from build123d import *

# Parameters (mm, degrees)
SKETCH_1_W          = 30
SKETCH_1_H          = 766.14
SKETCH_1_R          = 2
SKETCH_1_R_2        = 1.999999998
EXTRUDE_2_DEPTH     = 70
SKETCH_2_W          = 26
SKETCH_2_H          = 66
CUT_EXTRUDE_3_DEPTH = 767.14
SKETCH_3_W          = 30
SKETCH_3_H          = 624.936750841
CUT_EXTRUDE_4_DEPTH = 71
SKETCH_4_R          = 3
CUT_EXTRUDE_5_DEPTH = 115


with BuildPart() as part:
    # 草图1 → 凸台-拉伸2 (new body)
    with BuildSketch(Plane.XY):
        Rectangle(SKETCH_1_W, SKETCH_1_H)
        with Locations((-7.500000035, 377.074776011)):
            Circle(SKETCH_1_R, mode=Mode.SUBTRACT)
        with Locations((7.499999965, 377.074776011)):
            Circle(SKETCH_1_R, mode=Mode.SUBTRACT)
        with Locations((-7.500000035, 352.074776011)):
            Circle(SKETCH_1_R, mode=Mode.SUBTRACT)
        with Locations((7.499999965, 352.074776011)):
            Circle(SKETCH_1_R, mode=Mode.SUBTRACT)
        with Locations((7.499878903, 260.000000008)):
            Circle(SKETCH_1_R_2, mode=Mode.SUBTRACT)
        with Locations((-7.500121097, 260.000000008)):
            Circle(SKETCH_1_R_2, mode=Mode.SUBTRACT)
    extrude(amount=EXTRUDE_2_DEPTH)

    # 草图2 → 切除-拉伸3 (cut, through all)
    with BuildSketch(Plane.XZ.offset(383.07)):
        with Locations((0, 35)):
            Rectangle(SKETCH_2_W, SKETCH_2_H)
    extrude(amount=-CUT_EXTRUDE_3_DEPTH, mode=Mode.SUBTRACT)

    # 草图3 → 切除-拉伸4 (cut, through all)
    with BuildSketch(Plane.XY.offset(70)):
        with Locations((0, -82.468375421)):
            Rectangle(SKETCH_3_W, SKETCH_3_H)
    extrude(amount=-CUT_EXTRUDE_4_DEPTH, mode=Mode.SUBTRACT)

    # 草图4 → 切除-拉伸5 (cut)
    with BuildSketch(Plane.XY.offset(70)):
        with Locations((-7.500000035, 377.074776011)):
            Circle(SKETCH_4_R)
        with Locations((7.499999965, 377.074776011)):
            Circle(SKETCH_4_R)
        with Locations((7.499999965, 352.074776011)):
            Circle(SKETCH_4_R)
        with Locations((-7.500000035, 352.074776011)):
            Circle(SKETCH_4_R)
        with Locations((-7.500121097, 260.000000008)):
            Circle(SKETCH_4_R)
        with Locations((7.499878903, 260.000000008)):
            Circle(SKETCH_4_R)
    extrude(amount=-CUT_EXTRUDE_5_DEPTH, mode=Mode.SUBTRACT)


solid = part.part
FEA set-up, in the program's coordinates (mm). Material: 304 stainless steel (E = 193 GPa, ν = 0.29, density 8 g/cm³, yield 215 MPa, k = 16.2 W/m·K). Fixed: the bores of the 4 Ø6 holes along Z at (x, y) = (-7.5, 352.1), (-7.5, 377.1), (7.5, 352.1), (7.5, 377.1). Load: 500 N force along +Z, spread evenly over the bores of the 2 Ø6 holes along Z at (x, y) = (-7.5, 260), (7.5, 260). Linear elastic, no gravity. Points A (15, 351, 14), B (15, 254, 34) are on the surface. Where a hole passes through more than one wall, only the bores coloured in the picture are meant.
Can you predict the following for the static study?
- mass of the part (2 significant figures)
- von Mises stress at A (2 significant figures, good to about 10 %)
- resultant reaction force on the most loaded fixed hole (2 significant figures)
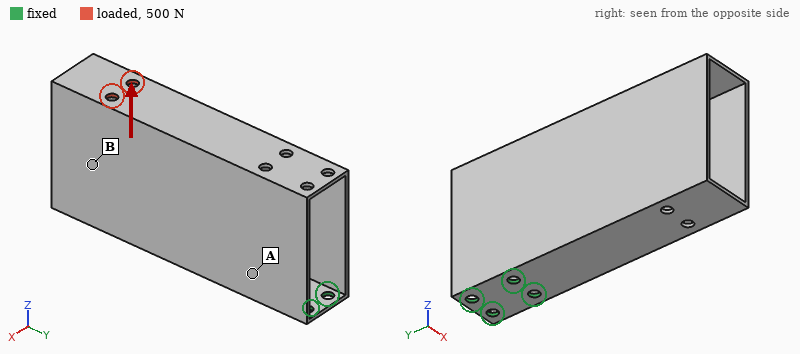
460 g
27 MPa
1.1 kN
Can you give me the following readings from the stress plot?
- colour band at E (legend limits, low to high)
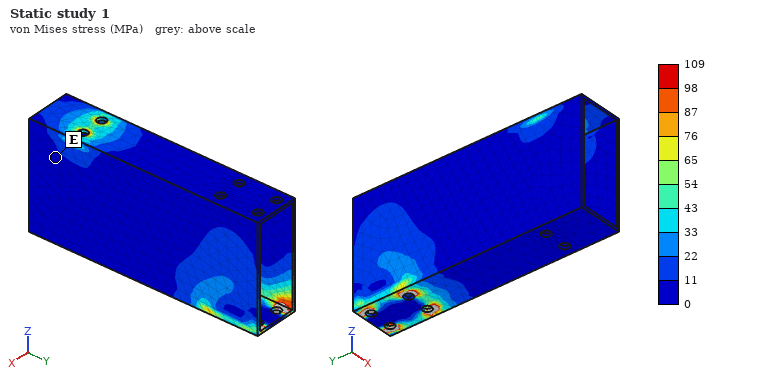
0 to 11 MPa
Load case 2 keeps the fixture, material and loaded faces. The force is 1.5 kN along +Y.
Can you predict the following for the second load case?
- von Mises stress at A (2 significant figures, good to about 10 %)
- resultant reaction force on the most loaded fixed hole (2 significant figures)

53 MPa
2.0 kN
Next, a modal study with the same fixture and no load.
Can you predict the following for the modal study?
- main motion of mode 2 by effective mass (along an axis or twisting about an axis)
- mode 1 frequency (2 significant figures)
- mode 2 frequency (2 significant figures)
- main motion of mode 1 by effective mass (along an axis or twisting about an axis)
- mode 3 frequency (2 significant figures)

along Z
320 Hz
580 Hz
along X
790 Hz
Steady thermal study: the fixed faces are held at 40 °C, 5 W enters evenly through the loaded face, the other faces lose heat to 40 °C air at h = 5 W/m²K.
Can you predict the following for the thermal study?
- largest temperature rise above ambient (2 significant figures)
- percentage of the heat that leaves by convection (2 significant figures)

73 K
88 %
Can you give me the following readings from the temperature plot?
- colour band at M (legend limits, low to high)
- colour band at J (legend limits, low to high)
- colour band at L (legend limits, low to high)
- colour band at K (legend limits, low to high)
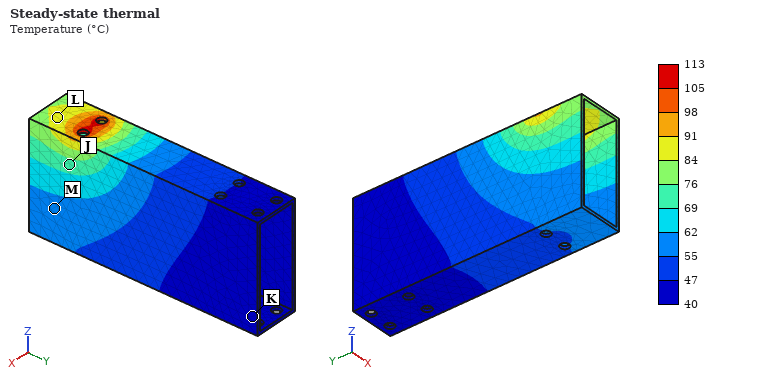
55 to 62 °C
69 to 76 °C
84 to 91 °C
40 to 47 °C
